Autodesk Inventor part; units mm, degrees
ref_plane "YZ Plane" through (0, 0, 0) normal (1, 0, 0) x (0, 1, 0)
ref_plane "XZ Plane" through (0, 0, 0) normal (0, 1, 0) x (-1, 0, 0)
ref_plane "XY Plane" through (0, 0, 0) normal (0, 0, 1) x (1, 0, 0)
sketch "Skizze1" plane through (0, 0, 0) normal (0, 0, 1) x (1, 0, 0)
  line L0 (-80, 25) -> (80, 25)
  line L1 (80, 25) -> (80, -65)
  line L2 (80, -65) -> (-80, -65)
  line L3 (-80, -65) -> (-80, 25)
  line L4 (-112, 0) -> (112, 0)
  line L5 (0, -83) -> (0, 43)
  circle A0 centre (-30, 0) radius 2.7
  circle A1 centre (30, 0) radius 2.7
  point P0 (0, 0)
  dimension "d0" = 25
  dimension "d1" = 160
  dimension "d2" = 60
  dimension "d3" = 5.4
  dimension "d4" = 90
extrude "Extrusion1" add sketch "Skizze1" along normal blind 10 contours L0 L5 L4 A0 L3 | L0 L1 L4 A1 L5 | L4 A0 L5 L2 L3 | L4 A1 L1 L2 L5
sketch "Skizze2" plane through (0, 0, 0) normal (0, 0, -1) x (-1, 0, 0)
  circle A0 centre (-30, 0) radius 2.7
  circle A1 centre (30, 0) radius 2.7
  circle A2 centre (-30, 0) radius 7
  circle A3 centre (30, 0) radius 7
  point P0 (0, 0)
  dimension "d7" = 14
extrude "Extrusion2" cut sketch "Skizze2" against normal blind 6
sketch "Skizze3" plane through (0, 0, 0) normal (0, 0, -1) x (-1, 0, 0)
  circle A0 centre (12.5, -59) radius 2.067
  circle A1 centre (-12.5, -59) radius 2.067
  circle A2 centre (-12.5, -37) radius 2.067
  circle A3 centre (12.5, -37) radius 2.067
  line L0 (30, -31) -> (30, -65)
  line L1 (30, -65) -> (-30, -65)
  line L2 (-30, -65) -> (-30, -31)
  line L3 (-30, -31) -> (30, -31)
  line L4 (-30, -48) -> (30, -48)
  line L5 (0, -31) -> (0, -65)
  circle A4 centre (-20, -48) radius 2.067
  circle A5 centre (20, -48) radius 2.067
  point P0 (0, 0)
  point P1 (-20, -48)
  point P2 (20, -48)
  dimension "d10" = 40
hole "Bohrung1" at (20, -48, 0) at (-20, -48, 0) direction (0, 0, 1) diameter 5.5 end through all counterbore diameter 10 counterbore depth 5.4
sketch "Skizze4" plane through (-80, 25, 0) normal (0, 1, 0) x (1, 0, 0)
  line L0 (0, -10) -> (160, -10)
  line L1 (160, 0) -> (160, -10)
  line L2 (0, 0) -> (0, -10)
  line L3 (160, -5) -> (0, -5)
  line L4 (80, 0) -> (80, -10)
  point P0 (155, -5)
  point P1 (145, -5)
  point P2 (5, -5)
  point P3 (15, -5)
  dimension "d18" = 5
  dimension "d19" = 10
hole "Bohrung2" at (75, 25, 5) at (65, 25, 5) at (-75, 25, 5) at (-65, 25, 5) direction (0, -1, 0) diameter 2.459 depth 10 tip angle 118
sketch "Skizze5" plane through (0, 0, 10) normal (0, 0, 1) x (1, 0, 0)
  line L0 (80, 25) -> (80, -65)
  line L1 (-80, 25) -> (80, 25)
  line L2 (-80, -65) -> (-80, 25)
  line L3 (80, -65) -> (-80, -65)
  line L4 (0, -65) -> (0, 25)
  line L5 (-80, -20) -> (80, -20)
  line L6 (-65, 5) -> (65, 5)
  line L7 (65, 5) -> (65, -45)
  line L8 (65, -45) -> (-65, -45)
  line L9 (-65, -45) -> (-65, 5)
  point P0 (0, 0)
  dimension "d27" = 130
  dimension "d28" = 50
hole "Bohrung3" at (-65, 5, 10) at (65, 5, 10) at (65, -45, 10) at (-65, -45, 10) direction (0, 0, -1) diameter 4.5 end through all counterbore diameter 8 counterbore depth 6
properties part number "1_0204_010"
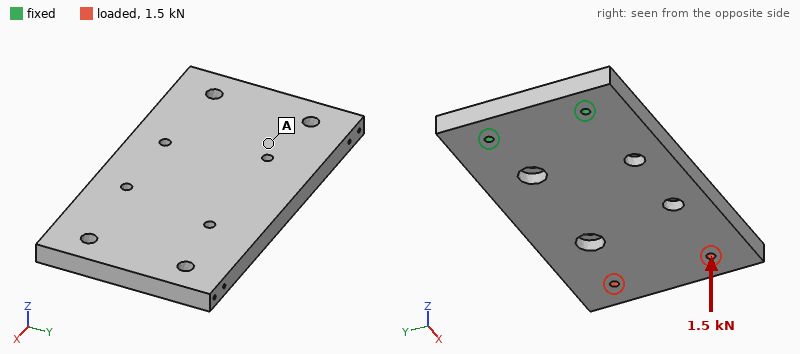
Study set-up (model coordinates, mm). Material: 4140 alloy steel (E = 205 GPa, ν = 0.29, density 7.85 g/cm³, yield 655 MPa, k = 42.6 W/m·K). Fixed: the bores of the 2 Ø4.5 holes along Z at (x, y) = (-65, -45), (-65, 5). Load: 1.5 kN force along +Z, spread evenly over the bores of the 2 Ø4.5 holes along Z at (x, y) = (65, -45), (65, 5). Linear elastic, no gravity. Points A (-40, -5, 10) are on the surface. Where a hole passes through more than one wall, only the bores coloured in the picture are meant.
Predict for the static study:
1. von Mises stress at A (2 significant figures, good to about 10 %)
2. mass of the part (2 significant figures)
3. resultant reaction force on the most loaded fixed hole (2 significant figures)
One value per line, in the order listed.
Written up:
92 MPa
1.1 kg
1.4 kN
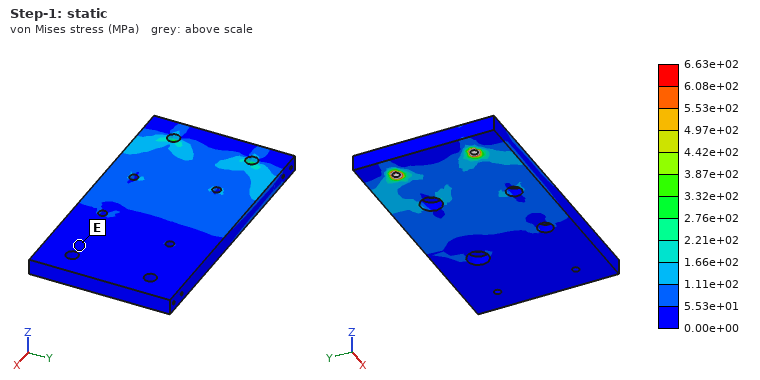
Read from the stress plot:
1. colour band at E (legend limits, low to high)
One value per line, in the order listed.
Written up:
0.00e+00 to 5.53e+01 MPa
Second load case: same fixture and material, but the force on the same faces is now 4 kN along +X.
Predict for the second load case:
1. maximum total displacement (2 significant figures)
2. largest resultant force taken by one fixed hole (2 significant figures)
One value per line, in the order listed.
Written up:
84 µm
2.0 kN
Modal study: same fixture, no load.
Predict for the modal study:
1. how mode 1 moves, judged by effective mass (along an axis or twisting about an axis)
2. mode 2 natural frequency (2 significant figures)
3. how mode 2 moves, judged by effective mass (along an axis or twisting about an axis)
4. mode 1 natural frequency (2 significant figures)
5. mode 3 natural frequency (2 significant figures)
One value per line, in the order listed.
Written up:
along Z
1200 Hz
twisting about X
250 Hz
1900 Hz
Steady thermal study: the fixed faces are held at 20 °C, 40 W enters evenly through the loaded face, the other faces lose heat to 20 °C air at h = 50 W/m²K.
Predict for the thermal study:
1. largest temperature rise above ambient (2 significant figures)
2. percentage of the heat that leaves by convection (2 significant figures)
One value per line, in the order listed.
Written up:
71 K
88 %
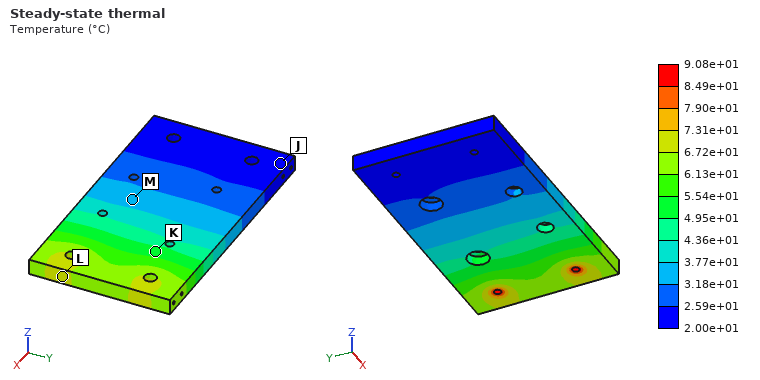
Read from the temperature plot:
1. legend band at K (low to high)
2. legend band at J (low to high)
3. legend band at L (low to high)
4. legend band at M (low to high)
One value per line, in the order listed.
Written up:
4.95e+01 to 5.54e+01 °C
2.00e+01 to 2.59e+01 °C
6.72e+01 to 7.31e+01 °C
3.18e+01 to 3.77e+01 °C
